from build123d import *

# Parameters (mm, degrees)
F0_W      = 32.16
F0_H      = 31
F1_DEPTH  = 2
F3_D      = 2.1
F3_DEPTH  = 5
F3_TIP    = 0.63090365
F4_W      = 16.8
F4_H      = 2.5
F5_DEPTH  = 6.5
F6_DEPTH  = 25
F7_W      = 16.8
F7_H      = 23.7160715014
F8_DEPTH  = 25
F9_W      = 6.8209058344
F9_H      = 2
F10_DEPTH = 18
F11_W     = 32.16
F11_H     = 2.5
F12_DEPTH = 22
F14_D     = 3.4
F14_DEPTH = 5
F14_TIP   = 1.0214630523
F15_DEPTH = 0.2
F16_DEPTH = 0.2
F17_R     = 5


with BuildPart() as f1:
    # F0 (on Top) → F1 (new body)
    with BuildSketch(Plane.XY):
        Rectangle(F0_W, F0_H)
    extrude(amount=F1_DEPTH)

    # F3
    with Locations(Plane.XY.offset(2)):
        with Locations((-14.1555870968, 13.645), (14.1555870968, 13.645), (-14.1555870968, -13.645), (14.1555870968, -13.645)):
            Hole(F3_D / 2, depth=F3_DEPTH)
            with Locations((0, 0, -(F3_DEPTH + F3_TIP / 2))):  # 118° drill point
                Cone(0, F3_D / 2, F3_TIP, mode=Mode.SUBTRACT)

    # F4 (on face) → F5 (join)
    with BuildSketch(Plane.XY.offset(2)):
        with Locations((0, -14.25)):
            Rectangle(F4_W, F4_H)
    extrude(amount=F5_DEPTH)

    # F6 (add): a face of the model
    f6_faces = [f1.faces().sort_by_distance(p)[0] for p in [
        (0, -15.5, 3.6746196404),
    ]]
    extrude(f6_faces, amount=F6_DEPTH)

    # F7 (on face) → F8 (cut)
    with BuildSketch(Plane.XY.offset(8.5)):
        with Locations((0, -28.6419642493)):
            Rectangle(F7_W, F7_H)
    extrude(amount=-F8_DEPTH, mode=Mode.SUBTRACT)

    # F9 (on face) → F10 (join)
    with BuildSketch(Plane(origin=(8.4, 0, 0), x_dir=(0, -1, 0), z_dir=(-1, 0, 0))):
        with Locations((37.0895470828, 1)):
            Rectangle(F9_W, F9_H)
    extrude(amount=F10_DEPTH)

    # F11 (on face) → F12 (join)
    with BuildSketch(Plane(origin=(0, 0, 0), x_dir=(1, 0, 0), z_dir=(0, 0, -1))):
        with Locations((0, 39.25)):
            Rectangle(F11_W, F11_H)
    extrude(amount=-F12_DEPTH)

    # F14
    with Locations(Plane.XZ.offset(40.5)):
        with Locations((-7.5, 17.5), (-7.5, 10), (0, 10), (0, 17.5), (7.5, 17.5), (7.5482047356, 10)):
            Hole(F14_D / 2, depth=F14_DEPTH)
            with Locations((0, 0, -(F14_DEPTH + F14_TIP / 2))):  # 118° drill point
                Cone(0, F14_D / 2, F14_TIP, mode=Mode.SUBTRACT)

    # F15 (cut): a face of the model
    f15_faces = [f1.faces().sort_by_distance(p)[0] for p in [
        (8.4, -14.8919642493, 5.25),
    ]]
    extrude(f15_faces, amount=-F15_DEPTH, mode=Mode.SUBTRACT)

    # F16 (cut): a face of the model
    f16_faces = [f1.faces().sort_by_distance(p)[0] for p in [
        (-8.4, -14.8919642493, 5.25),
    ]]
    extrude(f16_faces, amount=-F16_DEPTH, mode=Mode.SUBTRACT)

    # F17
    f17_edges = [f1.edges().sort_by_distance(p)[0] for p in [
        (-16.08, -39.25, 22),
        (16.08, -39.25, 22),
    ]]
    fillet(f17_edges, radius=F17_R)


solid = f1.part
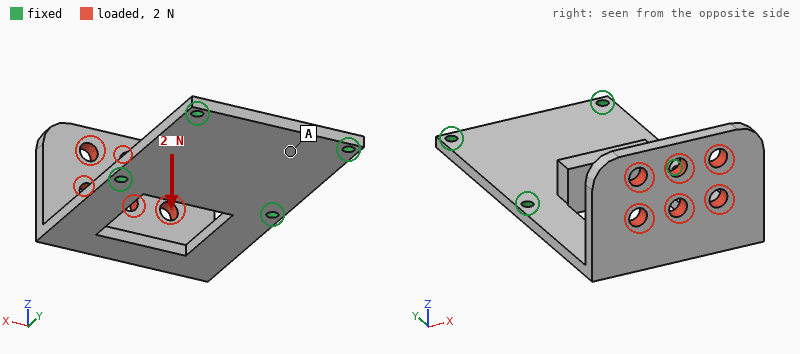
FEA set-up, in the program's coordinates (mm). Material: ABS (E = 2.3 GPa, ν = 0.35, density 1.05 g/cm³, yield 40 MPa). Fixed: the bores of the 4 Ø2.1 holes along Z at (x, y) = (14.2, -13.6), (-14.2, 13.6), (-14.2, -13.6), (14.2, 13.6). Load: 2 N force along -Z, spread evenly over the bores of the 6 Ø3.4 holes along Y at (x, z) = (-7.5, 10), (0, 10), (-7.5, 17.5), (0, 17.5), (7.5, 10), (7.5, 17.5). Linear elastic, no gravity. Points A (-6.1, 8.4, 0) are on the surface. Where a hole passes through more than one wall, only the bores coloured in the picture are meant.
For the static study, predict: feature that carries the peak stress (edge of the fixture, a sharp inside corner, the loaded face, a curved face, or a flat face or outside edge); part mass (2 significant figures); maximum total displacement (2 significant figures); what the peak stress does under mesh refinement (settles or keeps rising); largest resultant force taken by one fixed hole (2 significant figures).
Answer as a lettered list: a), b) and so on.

a) a sharp inside corner
b) 5.1 g
c) 0.73 mm
d) keeps rising
e) 1.2 N
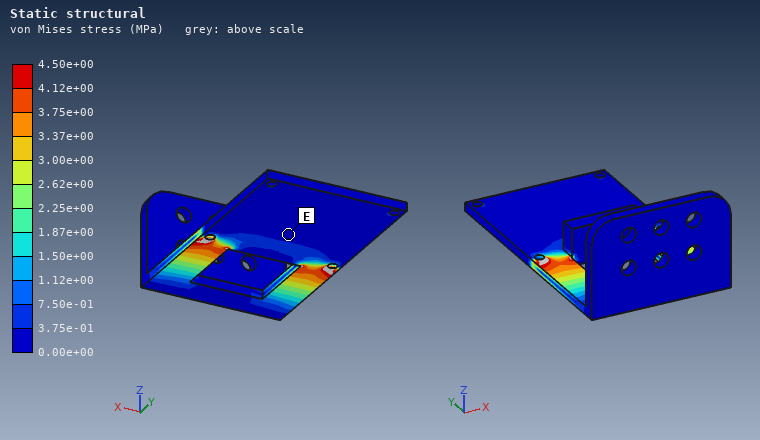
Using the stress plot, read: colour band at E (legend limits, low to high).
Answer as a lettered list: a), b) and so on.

a) 0.00e+00 to 3.75e-01 MPa
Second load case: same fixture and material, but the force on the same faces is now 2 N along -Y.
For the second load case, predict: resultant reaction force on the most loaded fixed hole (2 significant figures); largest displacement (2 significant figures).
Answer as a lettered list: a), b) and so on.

a) 0.99 N
b) 0.67 mm
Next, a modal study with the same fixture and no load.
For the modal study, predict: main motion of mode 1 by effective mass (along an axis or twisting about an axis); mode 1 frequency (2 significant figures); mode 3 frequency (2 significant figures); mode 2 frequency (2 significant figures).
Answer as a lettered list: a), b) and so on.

a) along Z
b) 200 Hz
c) 750 Hz
d) 470 Hz
